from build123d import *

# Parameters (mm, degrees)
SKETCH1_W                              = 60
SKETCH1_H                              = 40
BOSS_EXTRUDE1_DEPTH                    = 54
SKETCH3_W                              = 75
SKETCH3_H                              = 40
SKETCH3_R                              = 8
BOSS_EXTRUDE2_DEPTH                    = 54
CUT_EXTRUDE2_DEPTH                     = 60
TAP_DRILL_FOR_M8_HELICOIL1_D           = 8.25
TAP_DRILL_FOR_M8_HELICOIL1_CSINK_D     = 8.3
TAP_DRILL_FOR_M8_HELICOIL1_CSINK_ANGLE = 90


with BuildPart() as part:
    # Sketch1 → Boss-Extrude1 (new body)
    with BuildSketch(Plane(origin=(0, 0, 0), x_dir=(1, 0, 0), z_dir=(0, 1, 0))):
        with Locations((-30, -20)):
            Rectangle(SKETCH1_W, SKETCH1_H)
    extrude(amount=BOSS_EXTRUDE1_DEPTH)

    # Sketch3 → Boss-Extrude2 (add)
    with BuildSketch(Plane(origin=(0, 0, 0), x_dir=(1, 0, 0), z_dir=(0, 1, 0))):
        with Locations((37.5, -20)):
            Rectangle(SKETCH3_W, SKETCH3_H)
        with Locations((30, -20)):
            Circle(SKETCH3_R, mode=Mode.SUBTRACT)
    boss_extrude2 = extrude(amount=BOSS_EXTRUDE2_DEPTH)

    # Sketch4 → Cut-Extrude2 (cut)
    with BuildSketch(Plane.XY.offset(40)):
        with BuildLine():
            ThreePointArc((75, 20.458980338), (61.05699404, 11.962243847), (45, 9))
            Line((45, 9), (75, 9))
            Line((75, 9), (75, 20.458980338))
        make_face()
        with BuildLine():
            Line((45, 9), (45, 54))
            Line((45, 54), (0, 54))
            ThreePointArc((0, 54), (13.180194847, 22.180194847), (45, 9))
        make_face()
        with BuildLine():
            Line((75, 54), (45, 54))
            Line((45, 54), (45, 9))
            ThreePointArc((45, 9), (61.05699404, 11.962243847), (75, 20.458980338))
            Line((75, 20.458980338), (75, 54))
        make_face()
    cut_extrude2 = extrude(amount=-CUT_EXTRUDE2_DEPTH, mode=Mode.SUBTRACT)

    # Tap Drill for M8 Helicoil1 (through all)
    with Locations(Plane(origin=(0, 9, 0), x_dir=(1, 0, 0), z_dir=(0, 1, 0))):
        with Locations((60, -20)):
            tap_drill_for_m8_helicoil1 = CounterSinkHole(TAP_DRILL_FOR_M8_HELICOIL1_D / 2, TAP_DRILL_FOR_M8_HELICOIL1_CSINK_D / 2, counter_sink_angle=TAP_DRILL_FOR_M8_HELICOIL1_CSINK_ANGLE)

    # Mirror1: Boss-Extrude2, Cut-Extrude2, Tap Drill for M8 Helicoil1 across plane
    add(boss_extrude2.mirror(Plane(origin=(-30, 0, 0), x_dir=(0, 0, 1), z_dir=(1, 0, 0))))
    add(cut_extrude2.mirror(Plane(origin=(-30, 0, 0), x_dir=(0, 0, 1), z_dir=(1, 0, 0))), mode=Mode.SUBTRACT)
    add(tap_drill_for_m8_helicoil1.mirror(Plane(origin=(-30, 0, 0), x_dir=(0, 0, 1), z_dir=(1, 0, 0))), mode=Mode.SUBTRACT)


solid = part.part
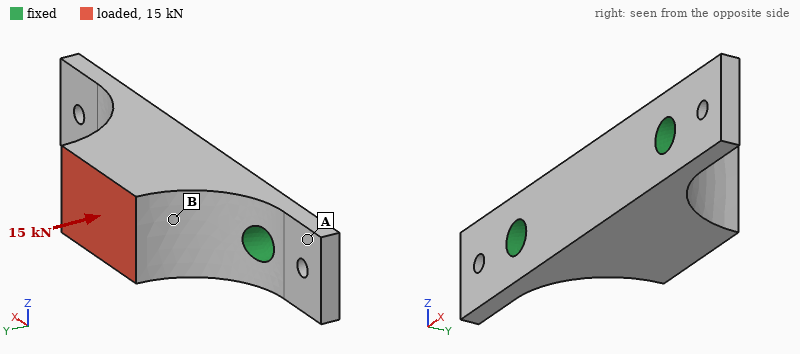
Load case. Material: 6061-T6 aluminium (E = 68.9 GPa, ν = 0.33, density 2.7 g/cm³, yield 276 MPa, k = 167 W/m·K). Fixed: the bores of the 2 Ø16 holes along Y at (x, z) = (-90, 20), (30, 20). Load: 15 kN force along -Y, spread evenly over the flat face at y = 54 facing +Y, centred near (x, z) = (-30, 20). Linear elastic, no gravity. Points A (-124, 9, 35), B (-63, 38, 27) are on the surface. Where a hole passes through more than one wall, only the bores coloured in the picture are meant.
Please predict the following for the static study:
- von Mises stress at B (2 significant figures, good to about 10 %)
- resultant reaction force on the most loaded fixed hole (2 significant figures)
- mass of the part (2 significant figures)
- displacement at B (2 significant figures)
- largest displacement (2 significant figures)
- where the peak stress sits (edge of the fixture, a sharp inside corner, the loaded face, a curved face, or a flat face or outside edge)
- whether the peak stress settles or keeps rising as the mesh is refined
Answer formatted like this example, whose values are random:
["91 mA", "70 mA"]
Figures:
["16 MPa", "9.3 kN", "570 g", "18 µm", "22 µm", "edge of the fixture", "keeps rising"]
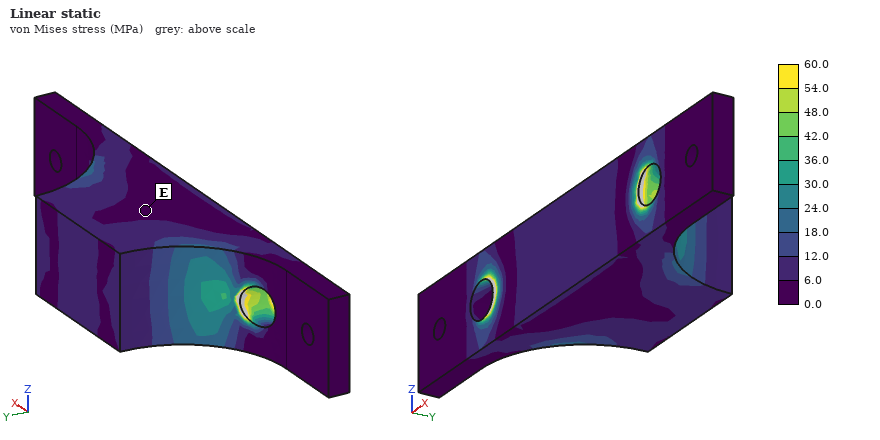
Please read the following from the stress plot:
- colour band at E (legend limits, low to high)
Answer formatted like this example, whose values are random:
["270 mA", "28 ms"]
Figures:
["0.0 to 6.0 MPa"]
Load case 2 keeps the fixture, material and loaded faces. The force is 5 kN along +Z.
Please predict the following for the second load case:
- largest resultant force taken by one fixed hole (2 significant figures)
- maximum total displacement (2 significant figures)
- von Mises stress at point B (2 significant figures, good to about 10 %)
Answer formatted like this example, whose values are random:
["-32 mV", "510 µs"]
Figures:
["2.5 kN", "90 µm", "13 MPa"]
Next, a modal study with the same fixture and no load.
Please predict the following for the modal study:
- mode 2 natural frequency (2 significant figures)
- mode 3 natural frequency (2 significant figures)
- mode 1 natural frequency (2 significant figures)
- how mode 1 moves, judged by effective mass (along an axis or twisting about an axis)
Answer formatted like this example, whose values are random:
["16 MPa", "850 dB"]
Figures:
["4700 Hz", "4700 Hz", "3300 Hz", "along Z"]
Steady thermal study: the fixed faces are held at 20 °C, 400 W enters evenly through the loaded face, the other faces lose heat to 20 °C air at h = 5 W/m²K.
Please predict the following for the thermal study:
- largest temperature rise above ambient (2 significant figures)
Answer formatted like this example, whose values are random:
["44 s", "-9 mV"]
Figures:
["80 K"]
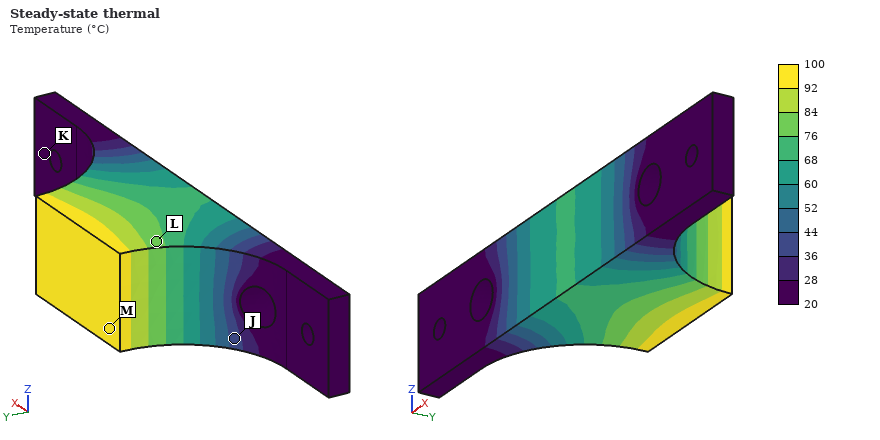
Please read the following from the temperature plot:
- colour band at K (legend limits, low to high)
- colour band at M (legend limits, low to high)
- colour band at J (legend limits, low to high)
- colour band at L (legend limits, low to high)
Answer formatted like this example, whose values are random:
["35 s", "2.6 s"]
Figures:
["20 to 28 °C", "92 to 100 °C", "36 to 44 °C", "76 to 84 °C"]
